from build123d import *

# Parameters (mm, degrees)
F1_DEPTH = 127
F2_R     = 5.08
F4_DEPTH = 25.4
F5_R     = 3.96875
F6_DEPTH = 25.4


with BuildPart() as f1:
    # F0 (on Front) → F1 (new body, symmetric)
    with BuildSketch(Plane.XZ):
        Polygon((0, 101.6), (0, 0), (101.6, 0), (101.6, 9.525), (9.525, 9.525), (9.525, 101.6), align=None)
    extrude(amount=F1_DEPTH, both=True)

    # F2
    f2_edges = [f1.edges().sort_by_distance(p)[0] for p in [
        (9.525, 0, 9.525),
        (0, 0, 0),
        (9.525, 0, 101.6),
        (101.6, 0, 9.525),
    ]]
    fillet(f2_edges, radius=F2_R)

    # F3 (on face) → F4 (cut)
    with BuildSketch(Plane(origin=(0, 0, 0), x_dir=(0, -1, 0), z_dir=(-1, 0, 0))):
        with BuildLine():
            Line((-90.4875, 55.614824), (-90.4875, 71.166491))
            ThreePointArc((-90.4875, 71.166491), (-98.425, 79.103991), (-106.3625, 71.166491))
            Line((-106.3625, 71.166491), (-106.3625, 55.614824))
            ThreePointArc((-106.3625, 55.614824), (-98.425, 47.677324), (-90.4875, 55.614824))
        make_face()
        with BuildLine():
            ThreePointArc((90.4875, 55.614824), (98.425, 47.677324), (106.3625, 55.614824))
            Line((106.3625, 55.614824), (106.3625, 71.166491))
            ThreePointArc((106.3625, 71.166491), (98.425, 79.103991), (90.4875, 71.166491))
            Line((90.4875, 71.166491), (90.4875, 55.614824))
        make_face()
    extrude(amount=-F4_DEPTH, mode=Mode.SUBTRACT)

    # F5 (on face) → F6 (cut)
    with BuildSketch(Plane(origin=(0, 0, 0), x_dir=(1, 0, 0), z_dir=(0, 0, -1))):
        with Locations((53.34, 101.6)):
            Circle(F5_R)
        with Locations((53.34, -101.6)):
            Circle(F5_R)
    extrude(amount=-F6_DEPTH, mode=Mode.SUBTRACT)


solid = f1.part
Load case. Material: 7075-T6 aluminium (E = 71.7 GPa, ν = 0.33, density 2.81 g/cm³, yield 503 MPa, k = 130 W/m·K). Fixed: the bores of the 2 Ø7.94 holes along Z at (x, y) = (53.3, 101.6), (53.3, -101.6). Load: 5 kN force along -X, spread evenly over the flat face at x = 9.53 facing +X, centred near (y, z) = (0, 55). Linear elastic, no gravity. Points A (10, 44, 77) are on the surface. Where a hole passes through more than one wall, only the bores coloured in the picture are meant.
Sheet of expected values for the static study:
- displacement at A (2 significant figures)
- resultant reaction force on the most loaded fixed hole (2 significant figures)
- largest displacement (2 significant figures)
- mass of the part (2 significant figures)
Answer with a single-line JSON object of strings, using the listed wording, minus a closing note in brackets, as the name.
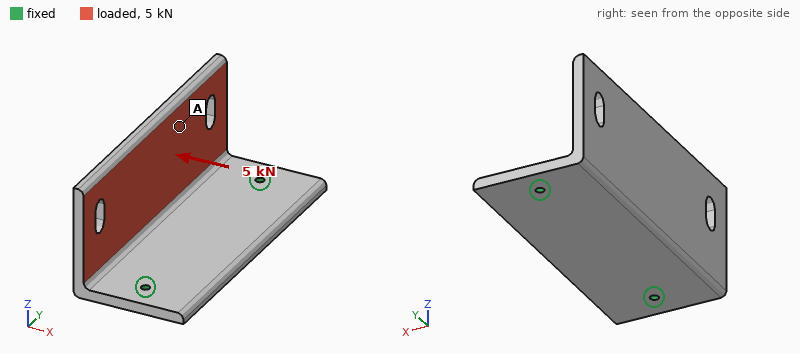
{"displacement at A": "1.2 mm", "resultant reaction force on the most loaded fixed hole": "2.5 kN", "largest displacement": "1.6 mm", "mass of the part": "1.3 kg"}
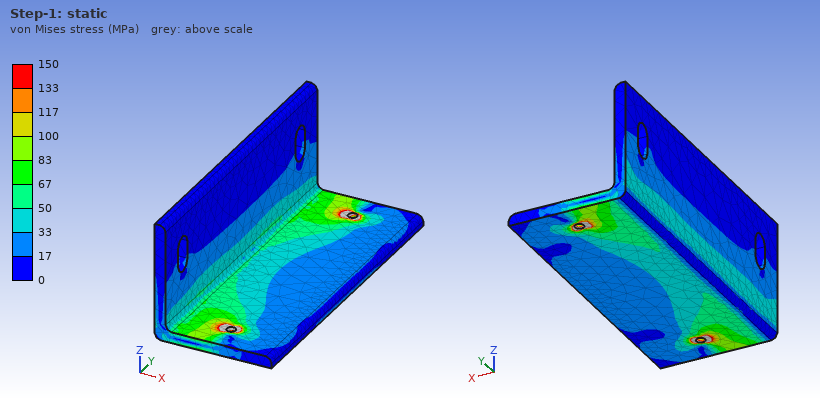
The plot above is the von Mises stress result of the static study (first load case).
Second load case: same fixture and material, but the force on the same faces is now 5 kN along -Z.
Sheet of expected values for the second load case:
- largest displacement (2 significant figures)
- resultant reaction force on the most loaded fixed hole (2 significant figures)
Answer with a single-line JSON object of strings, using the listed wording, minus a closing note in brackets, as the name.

{"largest displacement": "0.68 mm", "resultant reaction force on the most loaded fixed hole": "2.5 kN"}
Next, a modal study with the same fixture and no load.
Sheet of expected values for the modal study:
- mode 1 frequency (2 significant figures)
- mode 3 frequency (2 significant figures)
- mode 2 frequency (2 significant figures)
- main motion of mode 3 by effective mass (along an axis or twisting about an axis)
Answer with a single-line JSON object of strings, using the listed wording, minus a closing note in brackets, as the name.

{"mode 1 frequency": "400 Hz", "mode 3 frequency": "1100 Hz", "mode 2 frequency": "760 Hz", "main motion of mode 3 by effective mass": "along Z"}
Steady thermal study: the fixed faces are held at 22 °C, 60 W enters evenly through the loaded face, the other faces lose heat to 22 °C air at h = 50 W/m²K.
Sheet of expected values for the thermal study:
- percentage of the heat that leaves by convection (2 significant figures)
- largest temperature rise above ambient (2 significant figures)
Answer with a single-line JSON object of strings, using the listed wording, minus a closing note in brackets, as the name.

{"percentage of the heat that leaves by convection": "55 %", "largest temperature rise above ambient": "15 K"}
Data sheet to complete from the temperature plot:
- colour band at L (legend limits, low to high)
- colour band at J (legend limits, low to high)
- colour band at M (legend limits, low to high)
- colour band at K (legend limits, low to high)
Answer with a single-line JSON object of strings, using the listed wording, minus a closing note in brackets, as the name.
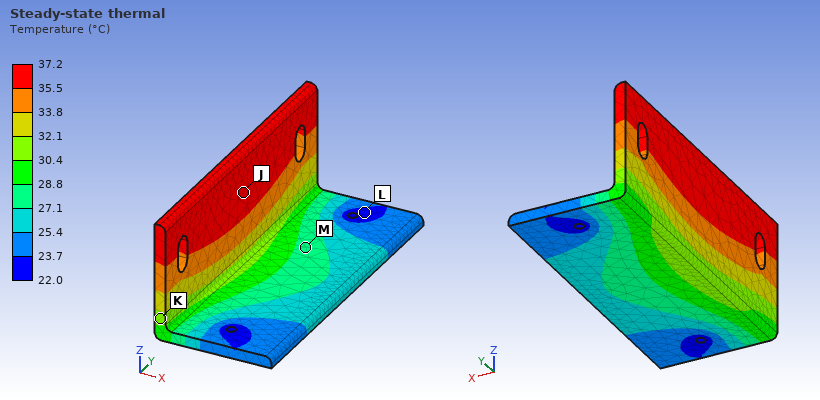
{"colour band at L": "22.0 to 23.7 °C", "colour band at J": "35.5 to 37.2 °C", "colour band at M": "27.1 to 28.8 °C", "colour band at K": "30.4 to 32.1 °C"}
